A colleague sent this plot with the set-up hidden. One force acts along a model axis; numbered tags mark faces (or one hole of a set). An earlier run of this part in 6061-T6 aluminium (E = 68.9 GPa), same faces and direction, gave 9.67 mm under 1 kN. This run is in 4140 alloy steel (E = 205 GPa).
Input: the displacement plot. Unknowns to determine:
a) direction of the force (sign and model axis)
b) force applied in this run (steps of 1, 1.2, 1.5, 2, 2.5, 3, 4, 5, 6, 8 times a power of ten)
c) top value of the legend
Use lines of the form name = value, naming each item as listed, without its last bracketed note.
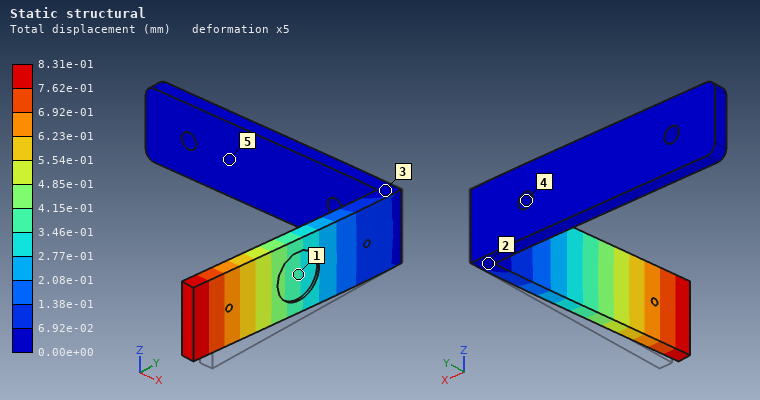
direction of the force = -X
force applied in this run = 250 N
top value of the legend = 8.31e-01 mm
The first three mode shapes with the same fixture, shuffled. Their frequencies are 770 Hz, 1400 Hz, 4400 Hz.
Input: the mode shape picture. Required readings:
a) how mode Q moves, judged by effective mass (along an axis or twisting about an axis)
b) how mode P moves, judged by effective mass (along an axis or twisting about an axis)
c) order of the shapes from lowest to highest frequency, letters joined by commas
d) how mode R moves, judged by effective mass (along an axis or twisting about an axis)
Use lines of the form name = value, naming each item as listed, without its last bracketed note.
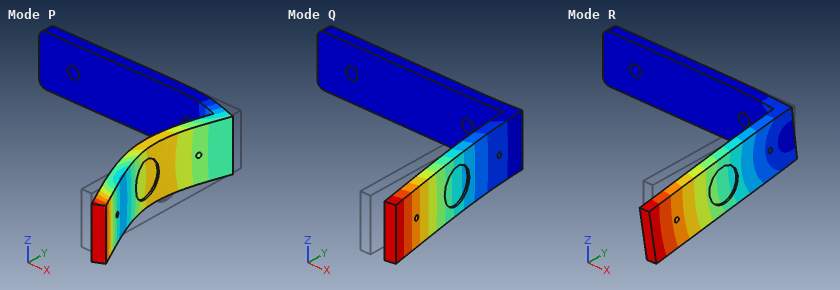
how mode Q moves, judged by effective mass = along X
how mode P moves, judged by effective mass = along Y
order of the shapes from lowest to highest frequency, letters joined by commas = Q, R, P
how mode R moves, judged by effective mass = along Z
